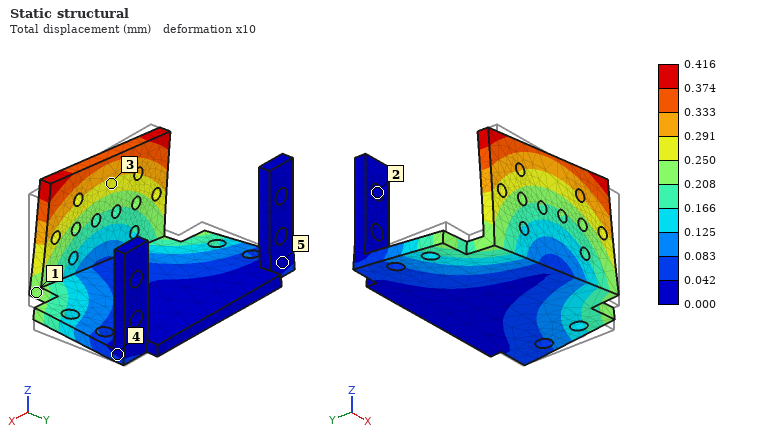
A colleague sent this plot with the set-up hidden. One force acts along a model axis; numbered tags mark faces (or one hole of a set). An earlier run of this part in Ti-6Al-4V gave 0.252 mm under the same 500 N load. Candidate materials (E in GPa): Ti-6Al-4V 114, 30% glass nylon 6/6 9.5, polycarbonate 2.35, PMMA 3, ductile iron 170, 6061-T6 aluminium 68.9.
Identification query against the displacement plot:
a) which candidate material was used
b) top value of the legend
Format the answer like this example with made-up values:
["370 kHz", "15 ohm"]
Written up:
["6061-T6 aluminium", "0.416 mm"]
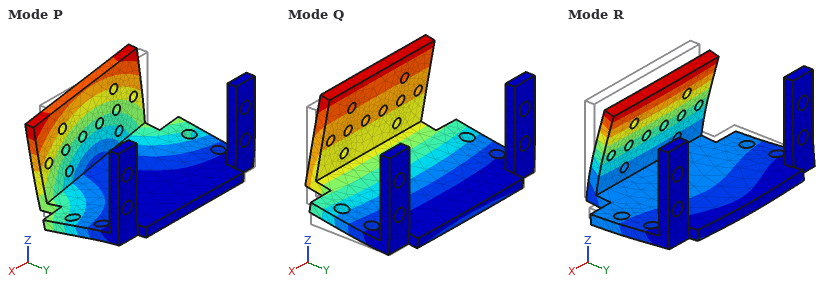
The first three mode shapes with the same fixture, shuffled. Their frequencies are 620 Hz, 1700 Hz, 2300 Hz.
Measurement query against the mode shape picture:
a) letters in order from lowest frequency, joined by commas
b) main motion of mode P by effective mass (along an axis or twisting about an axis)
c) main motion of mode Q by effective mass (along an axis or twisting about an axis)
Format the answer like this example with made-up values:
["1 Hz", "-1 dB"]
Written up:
["Q, P, R", "along X", "along Z"]
